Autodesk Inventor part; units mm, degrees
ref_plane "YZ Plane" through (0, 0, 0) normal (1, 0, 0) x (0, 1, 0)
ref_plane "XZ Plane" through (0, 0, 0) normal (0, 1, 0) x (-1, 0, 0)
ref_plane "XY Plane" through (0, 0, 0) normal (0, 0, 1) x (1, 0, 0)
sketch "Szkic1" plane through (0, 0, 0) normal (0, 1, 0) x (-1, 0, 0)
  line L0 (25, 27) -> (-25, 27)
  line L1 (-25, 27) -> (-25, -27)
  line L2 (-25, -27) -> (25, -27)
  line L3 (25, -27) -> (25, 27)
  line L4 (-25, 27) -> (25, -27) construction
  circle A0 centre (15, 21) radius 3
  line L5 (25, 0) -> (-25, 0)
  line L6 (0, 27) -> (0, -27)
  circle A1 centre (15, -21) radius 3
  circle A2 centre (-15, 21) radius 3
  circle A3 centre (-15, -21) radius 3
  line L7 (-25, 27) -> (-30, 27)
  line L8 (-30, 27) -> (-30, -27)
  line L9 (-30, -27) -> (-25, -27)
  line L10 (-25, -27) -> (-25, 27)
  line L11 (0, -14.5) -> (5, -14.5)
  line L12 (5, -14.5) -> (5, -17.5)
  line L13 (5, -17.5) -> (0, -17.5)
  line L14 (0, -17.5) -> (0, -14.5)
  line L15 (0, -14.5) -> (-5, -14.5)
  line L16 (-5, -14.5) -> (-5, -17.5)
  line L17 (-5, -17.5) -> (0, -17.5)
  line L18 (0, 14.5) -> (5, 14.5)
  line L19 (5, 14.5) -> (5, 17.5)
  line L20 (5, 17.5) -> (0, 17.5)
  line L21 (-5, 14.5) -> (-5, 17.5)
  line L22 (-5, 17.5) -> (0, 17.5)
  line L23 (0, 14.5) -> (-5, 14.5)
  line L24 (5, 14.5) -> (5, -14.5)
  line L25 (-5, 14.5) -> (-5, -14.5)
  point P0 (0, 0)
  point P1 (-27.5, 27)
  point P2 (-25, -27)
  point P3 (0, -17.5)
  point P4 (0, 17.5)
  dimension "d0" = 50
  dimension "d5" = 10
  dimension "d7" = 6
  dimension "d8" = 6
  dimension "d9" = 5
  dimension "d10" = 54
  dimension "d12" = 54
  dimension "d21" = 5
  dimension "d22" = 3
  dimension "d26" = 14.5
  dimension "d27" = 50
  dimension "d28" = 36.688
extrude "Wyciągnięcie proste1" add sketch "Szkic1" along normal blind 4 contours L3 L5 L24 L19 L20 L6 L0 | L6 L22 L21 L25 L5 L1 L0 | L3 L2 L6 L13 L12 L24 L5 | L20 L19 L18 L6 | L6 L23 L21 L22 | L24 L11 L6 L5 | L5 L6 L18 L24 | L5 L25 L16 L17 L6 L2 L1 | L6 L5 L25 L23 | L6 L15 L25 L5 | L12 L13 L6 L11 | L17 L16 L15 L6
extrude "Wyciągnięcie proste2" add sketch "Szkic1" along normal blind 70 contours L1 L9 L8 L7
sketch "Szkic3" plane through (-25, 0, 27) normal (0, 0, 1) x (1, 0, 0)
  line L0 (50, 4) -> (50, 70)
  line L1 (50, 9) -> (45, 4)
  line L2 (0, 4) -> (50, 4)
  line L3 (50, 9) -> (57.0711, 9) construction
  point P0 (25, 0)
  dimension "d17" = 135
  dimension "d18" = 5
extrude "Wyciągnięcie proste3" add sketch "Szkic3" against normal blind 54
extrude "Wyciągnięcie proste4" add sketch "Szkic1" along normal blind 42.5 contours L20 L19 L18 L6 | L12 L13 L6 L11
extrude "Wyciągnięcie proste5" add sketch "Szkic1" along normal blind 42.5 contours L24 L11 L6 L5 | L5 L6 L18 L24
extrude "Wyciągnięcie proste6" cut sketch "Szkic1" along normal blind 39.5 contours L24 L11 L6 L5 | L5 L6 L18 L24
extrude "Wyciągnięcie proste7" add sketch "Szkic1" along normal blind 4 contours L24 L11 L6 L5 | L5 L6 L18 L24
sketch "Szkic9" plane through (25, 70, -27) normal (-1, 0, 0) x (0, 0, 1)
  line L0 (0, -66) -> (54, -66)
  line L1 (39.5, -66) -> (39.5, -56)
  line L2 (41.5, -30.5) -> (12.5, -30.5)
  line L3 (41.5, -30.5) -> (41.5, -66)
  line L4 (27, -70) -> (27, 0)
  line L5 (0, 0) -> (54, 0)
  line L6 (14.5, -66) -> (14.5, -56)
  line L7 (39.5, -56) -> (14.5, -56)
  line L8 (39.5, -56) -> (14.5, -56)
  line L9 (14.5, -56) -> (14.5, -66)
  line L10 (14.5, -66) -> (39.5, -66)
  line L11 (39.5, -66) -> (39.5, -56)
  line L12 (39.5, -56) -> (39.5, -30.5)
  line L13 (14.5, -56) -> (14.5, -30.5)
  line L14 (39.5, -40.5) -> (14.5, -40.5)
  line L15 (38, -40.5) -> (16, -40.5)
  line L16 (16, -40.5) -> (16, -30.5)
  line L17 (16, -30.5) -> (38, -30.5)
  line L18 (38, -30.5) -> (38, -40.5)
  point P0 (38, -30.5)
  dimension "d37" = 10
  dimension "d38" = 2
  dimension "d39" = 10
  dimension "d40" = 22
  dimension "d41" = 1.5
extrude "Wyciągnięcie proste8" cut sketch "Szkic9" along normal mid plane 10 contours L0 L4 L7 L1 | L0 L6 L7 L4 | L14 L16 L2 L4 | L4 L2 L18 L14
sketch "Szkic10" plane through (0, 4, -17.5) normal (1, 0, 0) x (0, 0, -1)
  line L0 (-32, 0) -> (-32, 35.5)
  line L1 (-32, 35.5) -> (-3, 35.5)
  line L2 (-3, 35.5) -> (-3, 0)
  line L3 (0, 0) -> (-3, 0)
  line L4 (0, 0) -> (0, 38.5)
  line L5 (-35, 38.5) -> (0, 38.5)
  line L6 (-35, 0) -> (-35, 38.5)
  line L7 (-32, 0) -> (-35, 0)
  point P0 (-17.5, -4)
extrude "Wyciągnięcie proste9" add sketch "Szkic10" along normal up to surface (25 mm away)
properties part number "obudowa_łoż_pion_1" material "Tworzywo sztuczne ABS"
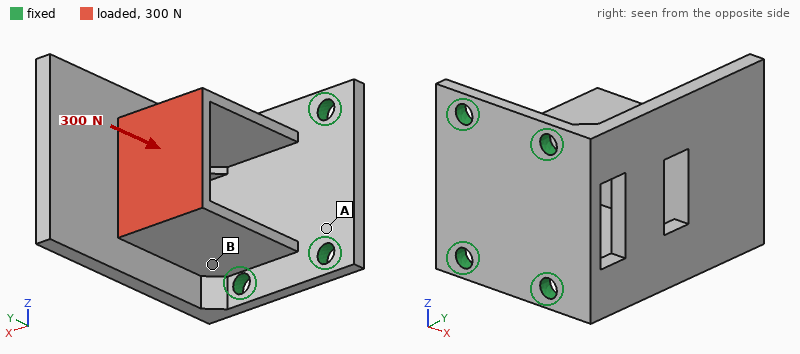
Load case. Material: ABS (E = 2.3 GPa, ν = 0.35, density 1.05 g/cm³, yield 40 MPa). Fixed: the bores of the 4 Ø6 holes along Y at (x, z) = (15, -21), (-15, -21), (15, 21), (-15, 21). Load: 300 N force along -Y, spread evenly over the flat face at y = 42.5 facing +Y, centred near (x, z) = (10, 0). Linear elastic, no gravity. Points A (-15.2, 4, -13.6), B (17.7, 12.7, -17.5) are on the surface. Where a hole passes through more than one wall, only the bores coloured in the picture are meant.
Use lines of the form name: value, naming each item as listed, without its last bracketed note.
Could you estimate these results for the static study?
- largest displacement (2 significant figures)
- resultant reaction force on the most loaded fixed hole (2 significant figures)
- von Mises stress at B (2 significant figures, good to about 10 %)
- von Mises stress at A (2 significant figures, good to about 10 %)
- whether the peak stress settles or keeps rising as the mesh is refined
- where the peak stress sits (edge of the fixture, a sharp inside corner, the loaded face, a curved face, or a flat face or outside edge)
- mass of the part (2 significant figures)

largest displacement: 0.38 mm
resultant reaction force on the most loaded fixed hole: 120 N
von Mises stress at B: 2.2 MPa
von Mises stress at A: 0.84 MPa
whether the peak stress settles or keeps rising as the mesh is refined: keeps rising
where the peak stress sits: edge of the fixture
mass of the part: 39 g
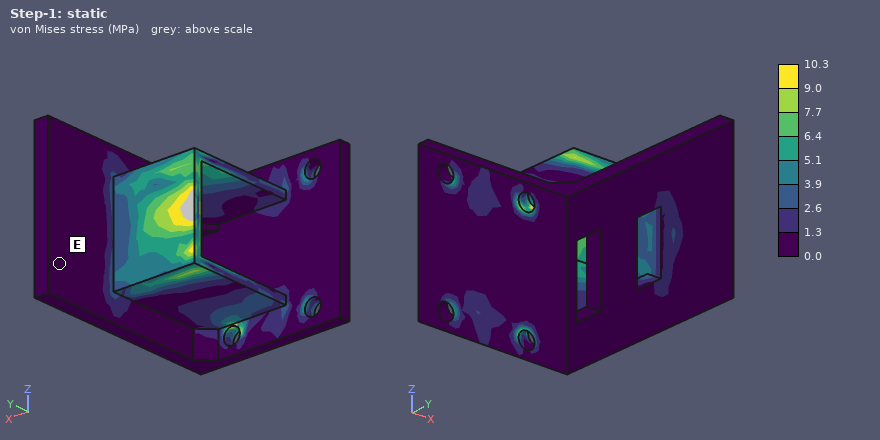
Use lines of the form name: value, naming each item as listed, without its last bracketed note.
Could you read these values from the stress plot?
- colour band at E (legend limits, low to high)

colour band at E: 0.0 to 1.3 MPa
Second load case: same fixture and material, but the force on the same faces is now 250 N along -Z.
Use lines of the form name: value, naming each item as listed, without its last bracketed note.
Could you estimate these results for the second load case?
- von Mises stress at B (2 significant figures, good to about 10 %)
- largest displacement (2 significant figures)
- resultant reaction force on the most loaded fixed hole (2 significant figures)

von Mises stress at B: 6.9 MPa
largest displacement: 1.2 mm
resultant reaction force on the most loaded fixed hole: 330 N
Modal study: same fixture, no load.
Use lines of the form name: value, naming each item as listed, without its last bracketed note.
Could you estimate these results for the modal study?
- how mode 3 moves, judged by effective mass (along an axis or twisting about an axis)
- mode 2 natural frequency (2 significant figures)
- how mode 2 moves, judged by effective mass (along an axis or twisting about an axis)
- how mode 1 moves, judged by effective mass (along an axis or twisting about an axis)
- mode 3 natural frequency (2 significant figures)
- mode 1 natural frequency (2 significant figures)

how mode 3 moves, judged by effective mass: along Z
mode 2 natural frequency: 740 Hz
how mode 2 moves, judged by effective mass: along Z
how mode 1 moves, judged by effective mass: along X
mode 3 natural frequency: 1400 Hz
mode 1 natural frequency: 650 Hz
